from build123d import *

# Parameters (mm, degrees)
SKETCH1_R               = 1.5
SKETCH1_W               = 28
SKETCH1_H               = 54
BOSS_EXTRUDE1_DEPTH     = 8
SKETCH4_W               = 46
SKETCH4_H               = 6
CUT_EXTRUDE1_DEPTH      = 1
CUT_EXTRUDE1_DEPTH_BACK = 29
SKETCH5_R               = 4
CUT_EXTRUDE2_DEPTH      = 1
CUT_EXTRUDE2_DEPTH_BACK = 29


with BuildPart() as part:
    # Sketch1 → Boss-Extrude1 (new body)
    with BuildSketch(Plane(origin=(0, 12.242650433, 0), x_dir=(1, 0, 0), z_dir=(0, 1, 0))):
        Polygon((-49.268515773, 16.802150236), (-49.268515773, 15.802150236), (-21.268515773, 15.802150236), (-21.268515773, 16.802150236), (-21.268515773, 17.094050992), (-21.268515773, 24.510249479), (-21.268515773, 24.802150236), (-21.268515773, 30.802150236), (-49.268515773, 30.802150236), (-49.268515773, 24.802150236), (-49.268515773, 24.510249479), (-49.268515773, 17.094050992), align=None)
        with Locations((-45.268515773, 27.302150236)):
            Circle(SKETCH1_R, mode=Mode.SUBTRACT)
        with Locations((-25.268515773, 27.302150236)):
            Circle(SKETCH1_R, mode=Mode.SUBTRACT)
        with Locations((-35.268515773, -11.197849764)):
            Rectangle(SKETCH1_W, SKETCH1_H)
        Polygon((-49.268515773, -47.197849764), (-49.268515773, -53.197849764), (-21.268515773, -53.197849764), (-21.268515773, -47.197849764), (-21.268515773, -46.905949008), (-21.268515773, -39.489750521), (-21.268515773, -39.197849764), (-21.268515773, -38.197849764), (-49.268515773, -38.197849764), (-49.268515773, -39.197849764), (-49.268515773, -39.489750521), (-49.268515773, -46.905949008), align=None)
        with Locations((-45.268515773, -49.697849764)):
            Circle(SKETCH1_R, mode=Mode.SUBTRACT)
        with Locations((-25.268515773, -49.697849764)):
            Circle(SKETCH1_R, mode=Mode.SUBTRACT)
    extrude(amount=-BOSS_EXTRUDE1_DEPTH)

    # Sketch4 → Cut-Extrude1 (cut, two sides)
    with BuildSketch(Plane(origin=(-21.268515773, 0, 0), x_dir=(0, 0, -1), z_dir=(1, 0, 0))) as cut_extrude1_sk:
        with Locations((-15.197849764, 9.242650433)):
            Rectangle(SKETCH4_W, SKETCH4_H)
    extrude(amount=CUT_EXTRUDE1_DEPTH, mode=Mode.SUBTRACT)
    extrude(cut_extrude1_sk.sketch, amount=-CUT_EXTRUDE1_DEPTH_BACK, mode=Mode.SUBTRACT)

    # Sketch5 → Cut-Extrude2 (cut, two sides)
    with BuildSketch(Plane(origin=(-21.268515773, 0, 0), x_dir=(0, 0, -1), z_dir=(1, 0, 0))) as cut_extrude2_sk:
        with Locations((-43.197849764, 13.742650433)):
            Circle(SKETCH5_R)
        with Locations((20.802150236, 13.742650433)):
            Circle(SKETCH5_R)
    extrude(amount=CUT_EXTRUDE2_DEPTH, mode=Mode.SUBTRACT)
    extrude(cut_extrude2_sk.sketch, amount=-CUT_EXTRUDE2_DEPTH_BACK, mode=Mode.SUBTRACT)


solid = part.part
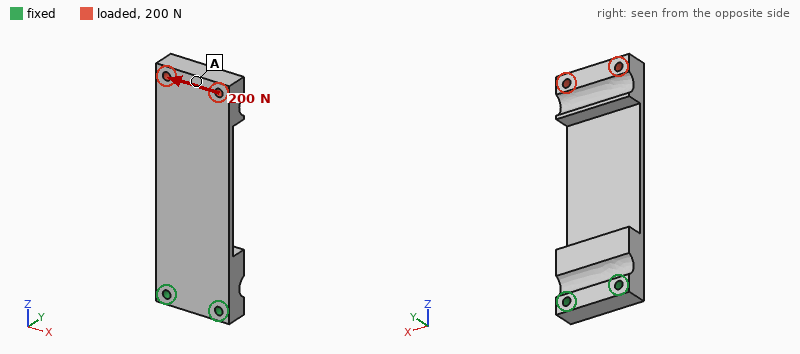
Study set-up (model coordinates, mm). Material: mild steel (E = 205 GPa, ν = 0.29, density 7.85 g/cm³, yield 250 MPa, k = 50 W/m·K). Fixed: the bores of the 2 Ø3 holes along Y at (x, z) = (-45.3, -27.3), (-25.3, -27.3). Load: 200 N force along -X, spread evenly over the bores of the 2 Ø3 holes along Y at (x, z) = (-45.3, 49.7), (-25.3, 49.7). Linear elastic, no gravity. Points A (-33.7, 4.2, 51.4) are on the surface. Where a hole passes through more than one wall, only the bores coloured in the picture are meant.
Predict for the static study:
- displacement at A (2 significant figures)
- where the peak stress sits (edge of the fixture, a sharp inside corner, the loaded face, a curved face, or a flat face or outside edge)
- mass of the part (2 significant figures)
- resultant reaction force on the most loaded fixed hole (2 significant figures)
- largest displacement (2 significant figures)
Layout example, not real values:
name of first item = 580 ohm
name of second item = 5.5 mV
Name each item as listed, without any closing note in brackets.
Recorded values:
displacement at A = 29 µm
where the peak stress sits = a flat face or outside edge
mass of the part = 79 g
resultant reaction force on the most loaded fixed hole = 740 N
largest displacement = 82 µm
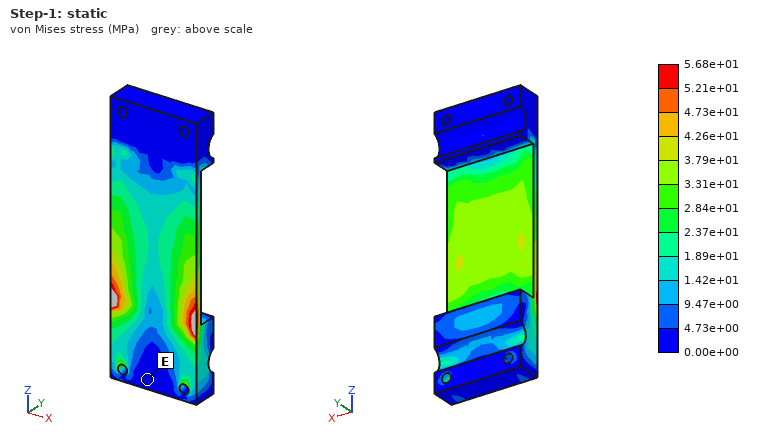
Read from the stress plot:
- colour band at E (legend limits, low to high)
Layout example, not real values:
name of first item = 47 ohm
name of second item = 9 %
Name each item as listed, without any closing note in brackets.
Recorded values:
colour band at E = 0.00e+00 to 4.73e+00 MPa
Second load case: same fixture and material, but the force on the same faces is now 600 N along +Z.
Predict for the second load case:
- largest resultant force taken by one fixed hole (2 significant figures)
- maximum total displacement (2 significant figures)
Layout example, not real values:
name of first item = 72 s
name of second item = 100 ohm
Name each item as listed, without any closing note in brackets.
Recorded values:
largest resultant force taken by one fixed hole = 300 N
maximum total displacement = 0.84 mm
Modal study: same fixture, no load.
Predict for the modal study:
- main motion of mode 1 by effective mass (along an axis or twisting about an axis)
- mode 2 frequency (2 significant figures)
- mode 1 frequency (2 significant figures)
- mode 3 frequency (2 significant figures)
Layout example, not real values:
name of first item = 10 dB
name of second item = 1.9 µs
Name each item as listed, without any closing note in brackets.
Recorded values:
main motion of mode 1 by effective mass = along Y
mode 2 frequency = 1300 Hz
mode 1 frequency = 260 Hz
mode 3 frequency = 2100 Hz
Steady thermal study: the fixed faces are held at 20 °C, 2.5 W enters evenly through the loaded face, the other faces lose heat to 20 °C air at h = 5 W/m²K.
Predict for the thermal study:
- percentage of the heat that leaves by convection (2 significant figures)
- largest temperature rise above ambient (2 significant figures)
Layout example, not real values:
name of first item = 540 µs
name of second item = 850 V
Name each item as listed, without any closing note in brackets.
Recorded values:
percentage of the heat that leaves by convection = 24 %
largest temperature rise above ambient = 43 K
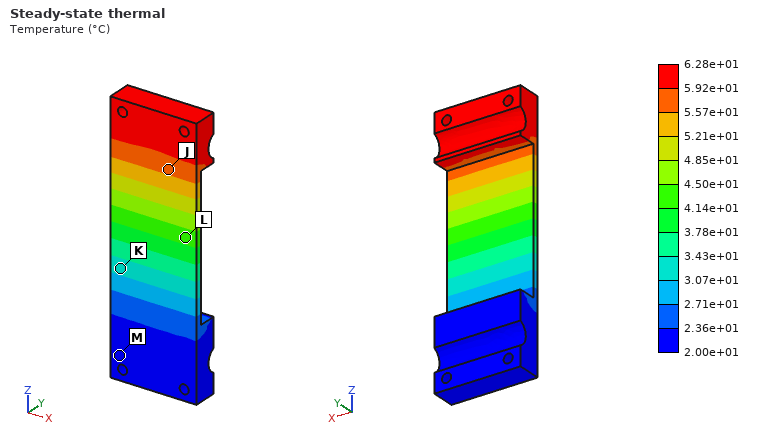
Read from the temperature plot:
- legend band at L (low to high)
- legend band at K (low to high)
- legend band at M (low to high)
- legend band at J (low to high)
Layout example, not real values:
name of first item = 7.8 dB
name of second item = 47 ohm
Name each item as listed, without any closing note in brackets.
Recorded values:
legend band at L = 4.14e+01 to 4.50e+01 °C
legend band at K = 3.07e+01 to 3.43e+01 °C
legend band at M = 2.00e+01 to 2.36e+01 °C
legend band at J = 5.57e+01 to 5.92e+01 °C
